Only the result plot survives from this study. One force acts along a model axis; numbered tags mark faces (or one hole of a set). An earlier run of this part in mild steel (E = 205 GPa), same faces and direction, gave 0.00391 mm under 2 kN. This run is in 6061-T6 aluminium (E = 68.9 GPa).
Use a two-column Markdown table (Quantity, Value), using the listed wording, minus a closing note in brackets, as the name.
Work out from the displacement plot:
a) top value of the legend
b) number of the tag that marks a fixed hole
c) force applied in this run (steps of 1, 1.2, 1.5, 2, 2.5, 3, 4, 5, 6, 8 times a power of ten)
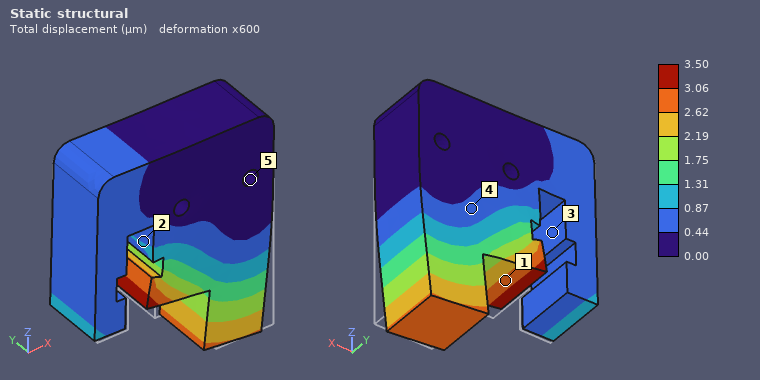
| Quantity | Value |
|---|---|
| top value of the legend | 3.50 µm |
| number of the tag that marks a fixed hole | 5 |
| force applied in this run | 600 N |
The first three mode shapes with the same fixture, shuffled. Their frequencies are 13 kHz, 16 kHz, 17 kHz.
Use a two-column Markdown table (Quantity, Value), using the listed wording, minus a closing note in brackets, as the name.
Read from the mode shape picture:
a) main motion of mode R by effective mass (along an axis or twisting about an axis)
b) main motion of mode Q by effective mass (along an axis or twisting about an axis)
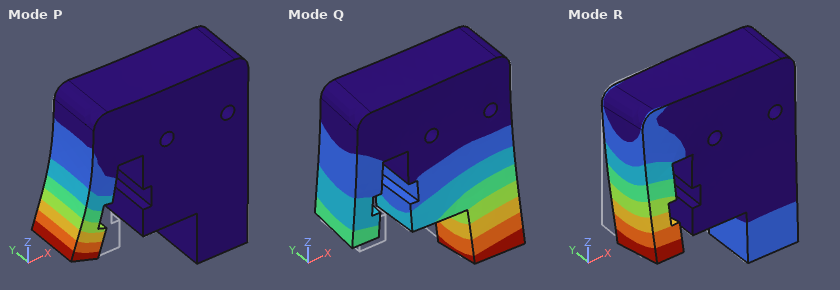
| Quantity | Value |
|---|---|
| main motion of mode R by effective mass | along Y |
| main motion of mode Q by effective mass | along Y |
